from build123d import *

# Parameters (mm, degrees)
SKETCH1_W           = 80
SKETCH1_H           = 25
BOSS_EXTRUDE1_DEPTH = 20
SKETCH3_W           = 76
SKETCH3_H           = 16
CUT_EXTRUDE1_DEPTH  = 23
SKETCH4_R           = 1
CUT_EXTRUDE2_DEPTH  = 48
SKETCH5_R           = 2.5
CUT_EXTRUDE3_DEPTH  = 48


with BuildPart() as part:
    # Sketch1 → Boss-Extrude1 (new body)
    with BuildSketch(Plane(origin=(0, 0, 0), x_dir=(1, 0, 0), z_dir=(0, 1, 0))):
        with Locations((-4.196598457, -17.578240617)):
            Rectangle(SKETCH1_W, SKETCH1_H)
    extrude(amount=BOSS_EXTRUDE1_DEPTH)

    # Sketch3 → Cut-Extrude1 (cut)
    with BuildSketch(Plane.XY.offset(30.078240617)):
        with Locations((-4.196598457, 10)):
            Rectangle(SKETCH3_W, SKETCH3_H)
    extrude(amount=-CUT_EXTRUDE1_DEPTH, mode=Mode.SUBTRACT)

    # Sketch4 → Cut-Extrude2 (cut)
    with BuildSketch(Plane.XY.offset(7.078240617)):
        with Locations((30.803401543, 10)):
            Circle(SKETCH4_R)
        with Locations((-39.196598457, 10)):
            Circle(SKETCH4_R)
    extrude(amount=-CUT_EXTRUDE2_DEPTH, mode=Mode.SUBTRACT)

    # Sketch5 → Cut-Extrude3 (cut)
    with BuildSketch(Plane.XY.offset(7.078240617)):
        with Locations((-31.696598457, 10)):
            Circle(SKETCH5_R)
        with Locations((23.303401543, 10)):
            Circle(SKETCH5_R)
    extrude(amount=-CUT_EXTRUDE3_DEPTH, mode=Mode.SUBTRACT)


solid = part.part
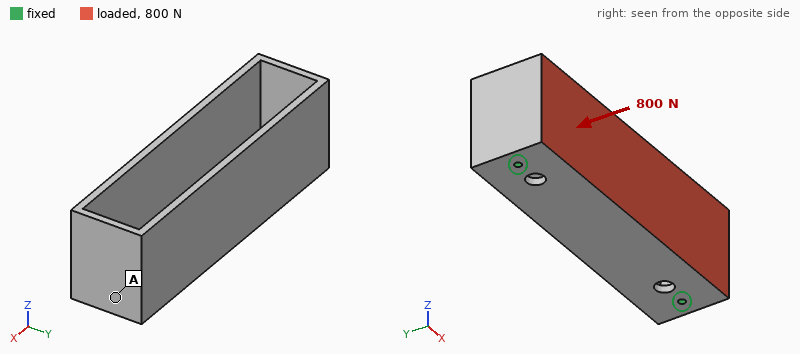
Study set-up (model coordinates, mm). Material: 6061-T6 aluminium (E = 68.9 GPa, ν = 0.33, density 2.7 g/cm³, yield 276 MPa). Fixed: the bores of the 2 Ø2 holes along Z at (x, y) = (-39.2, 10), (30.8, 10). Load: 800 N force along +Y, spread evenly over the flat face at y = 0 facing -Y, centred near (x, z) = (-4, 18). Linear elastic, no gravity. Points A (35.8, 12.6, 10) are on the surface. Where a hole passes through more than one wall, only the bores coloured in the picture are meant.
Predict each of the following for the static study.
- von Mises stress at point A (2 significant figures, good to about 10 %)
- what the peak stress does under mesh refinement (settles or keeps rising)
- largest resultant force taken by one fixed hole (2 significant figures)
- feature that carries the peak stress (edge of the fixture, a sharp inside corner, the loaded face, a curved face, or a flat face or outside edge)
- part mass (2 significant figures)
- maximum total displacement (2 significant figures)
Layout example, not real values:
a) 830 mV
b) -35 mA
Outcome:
a) 43 MPa
b) keeps rising
c) 400 N
d) edge of the fixture
e) 32 g
f) 0.69 mm
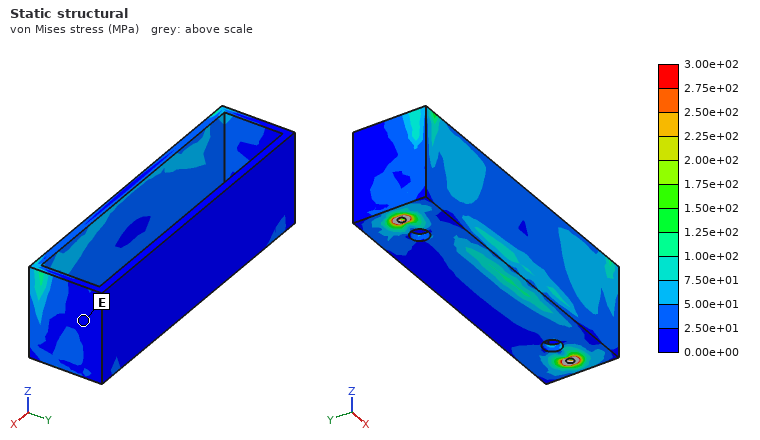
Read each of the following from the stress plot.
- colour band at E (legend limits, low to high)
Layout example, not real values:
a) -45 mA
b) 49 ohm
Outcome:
a) 0.00e+00 to 2.50e+01 MPa
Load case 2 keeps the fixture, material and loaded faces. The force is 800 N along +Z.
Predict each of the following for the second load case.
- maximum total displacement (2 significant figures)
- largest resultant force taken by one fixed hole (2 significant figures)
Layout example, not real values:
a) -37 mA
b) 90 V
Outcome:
a) 0.35 mm
b) 420 N
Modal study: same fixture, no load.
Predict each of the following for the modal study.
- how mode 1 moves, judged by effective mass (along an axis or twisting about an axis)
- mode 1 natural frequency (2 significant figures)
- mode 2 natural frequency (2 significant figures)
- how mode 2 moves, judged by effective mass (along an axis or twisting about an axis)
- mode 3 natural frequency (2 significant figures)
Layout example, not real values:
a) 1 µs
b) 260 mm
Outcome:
a) along Y
b) 1500 Hz
c) 2600 Hz
d) twisting about Z
e) 3000 Hz
